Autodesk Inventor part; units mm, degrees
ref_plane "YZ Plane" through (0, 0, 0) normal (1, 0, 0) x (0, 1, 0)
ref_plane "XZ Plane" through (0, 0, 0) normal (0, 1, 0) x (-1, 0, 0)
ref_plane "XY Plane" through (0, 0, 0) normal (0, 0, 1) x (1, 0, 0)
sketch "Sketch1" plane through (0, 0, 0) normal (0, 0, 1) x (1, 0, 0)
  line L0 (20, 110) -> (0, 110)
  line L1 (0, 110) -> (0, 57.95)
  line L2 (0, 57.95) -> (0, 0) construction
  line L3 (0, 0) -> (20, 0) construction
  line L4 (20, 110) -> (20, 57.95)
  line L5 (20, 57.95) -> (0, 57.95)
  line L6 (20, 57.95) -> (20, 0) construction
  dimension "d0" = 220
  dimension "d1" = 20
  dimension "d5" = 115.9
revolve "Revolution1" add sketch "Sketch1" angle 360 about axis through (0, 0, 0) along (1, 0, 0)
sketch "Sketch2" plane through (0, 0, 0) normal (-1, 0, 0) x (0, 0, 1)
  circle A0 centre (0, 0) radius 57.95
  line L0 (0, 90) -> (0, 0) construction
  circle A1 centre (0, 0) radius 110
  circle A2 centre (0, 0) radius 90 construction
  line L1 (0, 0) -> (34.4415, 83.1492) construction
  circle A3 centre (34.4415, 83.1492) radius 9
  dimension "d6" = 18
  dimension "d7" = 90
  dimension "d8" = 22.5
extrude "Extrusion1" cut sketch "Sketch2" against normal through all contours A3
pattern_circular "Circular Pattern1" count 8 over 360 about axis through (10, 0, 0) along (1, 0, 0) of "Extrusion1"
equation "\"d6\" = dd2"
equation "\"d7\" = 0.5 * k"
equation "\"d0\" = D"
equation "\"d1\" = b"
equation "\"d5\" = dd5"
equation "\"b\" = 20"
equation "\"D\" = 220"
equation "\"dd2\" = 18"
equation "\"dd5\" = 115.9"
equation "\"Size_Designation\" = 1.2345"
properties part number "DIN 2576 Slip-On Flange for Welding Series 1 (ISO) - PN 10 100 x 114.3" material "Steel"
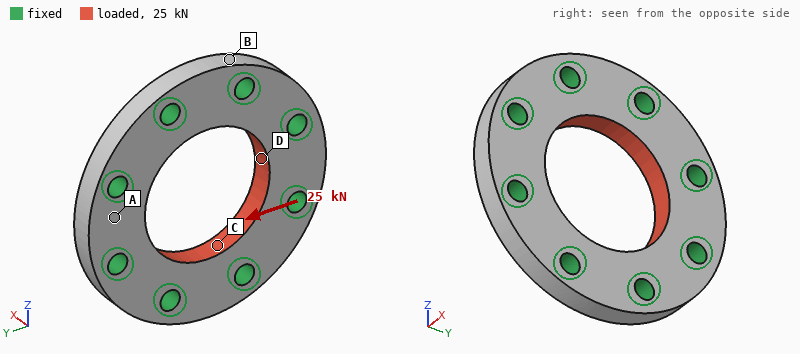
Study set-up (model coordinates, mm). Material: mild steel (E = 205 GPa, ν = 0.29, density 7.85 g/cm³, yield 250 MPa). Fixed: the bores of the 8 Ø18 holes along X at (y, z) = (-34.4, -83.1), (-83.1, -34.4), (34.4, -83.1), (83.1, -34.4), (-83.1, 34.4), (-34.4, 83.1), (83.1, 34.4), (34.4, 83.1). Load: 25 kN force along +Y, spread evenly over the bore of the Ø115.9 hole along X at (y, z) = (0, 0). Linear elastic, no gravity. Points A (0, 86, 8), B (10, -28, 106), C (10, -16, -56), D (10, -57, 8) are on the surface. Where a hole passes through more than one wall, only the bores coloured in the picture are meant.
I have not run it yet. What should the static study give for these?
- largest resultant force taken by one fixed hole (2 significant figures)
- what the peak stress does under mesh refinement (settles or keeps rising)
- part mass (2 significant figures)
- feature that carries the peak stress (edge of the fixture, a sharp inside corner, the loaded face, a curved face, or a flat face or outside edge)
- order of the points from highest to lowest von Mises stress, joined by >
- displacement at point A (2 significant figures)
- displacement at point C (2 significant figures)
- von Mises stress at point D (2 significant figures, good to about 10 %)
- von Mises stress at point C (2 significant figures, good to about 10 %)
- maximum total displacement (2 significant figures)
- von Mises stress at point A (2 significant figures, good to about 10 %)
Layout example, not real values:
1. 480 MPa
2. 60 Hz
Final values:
1. 4.0 kN
2. keeps rising
3. 4.0 kg
4. edge of the fixture
5. C > D > A > B
6. 0.44 µm
7. 0.79 µm
8. 3.1 MPa
9. 5.9 MPa
10. 0.84 µm
11. 1.7 MPa
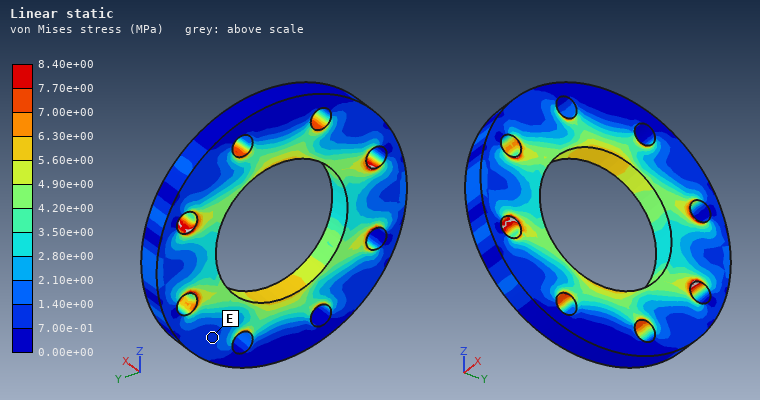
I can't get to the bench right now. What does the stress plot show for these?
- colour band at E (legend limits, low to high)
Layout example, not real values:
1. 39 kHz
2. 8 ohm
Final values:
1. 7.00e-01 to 1.40e+00 MPa
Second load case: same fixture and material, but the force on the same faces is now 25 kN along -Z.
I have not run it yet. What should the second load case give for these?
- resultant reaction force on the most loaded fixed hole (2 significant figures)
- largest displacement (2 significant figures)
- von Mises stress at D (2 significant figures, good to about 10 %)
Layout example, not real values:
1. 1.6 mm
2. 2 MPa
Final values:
1. 4.0 kN
2. 0.84 µm
3. 5.9 MPa
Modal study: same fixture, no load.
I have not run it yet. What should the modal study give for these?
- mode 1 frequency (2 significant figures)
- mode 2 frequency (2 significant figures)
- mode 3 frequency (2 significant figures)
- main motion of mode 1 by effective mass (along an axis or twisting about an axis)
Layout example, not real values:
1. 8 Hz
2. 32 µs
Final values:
1. 15 kHz
2. 15 kHz
3. 15 kHz
4. along X
